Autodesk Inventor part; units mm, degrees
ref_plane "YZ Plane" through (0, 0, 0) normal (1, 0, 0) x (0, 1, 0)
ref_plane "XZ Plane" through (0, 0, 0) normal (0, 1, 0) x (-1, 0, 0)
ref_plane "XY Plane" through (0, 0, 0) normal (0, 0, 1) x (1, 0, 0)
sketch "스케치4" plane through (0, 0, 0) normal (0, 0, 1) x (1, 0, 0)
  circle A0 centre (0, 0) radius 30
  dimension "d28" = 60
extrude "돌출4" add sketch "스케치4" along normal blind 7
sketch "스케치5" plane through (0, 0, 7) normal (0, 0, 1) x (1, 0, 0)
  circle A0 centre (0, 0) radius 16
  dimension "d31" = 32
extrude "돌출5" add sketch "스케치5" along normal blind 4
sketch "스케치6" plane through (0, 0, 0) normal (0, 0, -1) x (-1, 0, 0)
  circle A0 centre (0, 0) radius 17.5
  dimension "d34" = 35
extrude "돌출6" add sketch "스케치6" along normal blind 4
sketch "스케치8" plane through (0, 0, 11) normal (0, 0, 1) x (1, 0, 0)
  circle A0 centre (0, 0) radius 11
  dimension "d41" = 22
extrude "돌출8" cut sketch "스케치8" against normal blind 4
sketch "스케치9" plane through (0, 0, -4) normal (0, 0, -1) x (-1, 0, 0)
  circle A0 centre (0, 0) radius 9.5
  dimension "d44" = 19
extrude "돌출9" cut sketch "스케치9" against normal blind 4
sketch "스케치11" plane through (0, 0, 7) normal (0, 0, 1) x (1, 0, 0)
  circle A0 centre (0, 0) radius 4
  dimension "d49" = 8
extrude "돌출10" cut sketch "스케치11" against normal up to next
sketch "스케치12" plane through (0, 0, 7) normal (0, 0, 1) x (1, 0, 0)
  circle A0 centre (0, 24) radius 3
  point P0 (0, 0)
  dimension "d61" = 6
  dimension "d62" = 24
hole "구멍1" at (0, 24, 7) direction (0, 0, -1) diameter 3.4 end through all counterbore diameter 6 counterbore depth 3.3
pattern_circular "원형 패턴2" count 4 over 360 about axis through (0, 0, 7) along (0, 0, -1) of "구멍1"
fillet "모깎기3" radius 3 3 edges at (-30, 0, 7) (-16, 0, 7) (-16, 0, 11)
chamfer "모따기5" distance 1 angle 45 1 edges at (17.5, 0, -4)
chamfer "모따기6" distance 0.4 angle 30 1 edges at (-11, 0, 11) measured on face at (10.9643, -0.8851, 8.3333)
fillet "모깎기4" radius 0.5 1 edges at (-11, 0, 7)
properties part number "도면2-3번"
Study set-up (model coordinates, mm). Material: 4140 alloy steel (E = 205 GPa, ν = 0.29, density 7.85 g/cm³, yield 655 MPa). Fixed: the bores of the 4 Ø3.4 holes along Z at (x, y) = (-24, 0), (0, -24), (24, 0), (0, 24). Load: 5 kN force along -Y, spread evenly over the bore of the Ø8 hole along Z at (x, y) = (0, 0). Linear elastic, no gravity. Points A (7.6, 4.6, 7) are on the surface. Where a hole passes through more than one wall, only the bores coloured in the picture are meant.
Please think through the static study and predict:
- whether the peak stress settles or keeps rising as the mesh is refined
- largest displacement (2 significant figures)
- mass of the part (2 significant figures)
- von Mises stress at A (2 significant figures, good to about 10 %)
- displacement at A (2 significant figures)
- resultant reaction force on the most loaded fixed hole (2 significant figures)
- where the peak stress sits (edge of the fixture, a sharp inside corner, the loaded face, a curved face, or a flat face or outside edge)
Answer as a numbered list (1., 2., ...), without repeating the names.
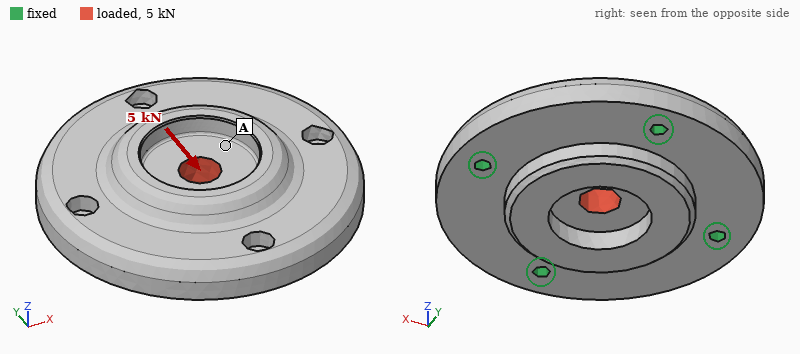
1. keeps rising
2. 2.4 µm
3. 180 g
4. 11 MPa
5. 1.6 µm
6. 1.5 kN
7. edge of the fixture
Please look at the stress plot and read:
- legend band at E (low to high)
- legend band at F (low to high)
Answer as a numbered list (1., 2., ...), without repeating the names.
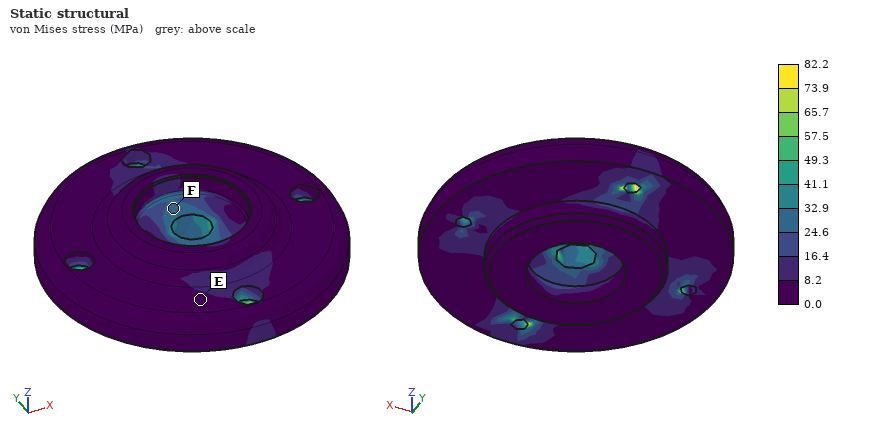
1. 0.0 to 8.2 MPa
2. 24.6 to 32.9 MPa
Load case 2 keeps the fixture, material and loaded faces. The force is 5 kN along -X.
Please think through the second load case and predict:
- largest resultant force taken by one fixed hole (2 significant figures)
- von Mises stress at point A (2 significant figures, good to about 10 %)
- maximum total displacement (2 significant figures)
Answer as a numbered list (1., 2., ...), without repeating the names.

1. 1.5 kN
2. 20 MPa
3. 2.4 µm
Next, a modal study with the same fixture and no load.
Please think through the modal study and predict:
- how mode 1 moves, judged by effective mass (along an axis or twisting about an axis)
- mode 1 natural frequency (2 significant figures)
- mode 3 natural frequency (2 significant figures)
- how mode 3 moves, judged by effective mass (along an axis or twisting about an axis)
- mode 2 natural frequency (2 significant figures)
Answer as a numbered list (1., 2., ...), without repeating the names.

1. along Z
2. 16 kHz
3. 18 kHz
4. twisting about Y
5. 17 kHz
